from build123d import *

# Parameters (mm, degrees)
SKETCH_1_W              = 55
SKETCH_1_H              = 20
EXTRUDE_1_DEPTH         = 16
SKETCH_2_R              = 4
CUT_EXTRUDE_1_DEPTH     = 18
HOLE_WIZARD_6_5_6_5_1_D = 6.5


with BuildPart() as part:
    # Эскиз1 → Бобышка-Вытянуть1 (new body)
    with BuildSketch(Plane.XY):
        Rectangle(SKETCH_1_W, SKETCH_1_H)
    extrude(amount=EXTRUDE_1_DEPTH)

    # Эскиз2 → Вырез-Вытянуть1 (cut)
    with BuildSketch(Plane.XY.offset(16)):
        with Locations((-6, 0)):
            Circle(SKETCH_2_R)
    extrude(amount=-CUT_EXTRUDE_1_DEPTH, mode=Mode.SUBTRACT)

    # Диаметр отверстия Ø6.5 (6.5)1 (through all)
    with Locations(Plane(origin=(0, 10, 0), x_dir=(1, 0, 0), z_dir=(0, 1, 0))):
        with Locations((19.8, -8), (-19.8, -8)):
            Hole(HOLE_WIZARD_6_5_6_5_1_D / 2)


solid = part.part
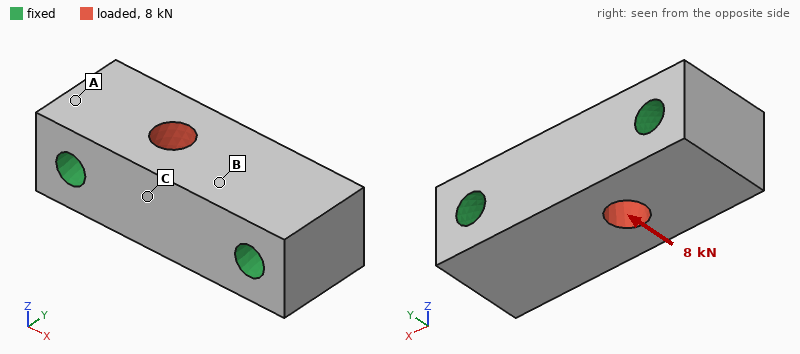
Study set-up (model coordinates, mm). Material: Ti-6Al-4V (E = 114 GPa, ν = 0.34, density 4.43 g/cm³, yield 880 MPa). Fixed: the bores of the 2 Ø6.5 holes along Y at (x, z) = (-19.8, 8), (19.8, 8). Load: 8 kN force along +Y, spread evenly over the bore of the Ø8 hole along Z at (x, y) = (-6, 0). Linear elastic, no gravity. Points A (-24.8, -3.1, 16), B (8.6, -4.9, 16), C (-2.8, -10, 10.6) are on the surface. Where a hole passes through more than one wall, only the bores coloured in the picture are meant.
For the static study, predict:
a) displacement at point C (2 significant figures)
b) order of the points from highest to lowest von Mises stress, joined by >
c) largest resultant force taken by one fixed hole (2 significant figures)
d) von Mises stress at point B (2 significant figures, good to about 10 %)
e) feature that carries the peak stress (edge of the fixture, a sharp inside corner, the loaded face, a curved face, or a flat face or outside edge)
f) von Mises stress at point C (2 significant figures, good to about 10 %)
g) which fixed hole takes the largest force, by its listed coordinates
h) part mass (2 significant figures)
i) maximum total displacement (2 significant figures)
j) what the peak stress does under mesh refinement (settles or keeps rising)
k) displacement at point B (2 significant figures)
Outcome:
6.5 µm
C > B > A
5.3 kN
18 MPa
edge of the fixture
38 MPa
(-19.8, 8)
69 g
7.7 µm
keeps rising
3.2 µm
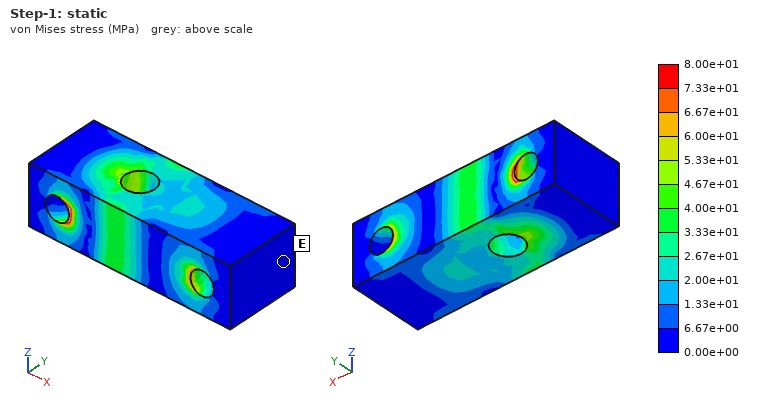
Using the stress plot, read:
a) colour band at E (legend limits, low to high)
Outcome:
0.00e+00 to 6.67e+00 MPa
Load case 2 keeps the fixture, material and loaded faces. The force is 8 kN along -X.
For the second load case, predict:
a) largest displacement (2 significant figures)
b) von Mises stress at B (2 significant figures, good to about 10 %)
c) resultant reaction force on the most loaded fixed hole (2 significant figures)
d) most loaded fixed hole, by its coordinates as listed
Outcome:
2.5 µm
9.4 MPa
5.0 kN
(-19.8, 8)
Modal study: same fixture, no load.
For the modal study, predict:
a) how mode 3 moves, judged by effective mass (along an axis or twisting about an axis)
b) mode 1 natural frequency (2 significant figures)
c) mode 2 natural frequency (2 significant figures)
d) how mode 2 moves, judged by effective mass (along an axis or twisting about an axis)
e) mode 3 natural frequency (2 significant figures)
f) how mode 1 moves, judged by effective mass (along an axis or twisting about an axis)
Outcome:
twisting about X
30 kHz
34 kHz
along Y
38 kHz
along Z
